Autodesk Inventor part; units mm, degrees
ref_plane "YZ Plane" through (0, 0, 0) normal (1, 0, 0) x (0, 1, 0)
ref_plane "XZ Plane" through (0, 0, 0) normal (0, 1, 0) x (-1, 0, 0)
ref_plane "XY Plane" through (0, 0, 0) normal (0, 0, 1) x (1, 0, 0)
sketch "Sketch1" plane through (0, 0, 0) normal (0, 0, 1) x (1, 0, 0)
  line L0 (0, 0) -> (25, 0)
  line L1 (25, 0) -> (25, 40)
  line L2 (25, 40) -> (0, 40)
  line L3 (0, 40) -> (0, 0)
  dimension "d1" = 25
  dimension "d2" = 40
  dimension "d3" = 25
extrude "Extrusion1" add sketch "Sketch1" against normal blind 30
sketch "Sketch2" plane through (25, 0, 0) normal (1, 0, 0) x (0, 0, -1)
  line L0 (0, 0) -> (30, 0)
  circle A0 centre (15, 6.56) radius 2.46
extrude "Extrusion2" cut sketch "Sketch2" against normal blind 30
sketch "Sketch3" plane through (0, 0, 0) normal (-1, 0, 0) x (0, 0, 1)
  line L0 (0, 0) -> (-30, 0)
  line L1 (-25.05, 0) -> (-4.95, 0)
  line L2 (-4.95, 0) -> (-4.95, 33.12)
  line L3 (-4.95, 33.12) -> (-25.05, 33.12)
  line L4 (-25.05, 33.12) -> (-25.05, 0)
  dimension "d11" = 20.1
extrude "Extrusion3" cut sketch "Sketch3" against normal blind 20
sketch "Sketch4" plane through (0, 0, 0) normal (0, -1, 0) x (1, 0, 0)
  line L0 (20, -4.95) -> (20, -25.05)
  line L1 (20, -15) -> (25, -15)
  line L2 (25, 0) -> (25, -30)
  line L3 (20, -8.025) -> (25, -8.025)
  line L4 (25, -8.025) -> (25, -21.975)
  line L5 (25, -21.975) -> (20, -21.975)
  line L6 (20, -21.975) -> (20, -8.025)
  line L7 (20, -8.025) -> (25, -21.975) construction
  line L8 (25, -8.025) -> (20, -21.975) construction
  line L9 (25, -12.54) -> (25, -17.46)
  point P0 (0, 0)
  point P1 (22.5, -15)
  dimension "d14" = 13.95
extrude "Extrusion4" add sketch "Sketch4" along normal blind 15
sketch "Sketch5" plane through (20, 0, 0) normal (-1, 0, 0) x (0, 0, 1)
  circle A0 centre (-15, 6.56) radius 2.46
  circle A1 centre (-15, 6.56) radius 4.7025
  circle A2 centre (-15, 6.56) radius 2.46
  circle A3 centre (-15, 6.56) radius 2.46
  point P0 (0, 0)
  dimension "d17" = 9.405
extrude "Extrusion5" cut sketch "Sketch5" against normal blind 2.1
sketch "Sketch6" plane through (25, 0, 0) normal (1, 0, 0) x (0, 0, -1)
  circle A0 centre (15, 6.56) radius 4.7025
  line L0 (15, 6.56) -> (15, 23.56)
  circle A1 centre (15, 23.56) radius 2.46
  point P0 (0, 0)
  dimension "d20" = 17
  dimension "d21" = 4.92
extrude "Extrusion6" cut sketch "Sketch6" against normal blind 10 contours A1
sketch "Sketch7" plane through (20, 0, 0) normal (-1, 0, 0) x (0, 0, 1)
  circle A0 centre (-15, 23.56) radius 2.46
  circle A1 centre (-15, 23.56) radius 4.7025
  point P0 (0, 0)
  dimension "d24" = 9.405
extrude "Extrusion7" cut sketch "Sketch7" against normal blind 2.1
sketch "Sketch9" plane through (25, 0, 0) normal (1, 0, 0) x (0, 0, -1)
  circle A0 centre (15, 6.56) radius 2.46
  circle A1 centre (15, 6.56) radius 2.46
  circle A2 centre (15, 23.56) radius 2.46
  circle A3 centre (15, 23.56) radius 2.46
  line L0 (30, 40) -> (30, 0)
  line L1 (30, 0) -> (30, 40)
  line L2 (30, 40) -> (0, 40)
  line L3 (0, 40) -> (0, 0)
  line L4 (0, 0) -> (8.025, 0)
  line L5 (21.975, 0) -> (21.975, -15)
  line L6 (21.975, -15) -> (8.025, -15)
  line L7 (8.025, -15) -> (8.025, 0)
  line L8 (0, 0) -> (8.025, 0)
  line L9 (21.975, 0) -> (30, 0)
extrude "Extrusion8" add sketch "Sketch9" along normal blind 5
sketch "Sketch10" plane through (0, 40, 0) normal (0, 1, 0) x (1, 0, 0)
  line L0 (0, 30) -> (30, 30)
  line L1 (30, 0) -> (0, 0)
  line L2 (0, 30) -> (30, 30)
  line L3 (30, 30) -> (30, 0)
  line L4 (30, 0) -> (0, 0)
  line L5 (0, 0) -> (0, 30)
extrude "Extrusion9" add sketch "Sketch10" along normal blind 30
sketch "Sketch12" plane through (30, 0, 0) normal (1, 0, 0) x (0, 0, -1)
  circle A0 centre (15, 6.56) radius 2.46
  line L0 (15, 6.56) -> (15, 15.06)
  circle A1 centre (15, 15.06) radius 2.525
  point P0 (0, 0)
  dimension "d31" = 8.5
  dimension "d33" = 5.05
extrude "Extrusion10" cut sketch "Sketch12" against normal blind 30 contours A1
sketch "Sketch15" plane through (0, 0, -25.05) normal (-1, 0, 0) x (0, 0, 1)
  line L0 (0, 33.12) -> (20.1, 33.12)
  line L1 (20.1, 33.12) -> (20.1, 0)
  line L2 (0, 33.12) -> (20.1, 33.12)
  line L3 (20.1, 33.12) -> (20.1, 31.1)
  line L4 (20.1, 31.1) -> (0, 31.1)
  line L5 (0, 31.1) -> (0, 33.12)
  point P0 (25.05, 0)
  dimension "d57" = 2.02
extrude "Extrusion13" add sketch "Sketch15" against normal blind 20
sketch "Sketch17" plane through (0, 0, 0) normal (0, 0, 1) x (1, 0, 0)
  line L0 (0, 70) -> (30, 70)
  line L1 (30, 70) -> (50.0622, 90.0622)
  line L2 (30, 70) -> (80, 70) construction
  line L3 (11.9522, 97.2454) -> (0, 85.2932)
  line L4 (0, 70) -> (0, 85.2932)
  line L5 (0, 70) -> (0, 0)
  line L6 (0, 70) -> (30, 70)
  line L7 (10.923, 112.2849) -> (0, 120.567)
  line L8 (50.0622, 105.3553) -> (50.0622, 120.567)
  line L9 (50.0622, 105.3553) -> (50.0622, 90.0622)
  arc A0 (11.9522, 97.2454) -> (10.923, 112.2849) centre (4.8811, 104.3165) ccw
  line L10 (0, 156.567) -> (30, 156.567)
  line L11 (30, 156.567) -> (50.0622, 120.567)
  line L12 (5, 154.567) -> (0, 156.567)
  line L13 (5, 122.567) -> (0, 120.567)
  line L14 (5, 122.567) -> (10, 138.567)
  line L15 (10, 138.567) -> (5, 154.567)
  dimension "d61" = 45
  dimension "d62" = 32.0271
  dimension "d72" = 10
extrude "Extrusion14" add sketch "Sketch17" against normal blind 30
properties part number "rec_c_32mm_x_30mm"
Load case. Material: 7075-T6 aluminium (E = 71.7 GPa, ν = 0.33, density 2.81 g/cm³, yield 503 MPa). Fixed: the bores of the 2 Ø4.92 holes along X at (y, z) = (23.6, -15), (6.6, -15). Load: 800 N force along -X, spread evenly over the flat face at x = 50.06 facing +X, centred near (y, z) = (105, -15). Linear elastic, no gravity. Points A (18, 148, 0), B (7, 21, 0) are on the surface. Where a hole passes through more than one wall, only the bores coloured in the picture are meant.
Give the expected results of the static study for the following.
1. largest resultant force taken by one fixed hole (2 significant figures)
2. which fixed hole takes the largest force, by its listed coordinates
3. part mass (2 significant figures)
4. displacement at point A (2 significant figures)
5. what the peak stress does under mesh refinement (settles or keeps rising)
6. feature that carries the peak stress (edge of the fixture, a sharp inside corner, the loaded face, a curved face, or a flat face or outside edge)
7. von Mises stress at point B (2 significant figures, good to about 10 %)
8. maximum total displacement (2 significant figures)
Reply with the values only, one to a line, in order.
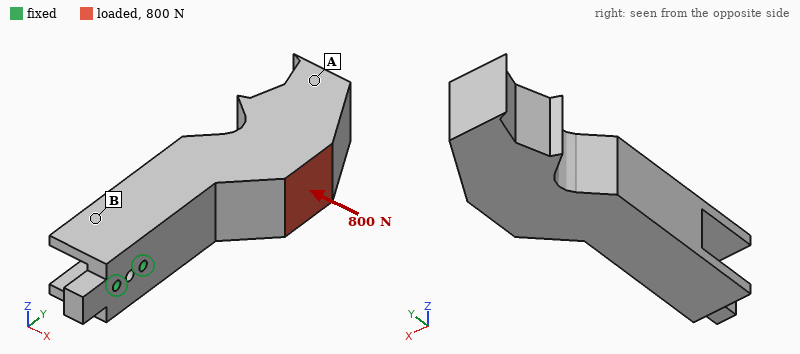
3.4 kN
(23.6, -15)
420 g
0.22 mm
keeps rising
edge of the fixture
17 MPa
0.24 mm
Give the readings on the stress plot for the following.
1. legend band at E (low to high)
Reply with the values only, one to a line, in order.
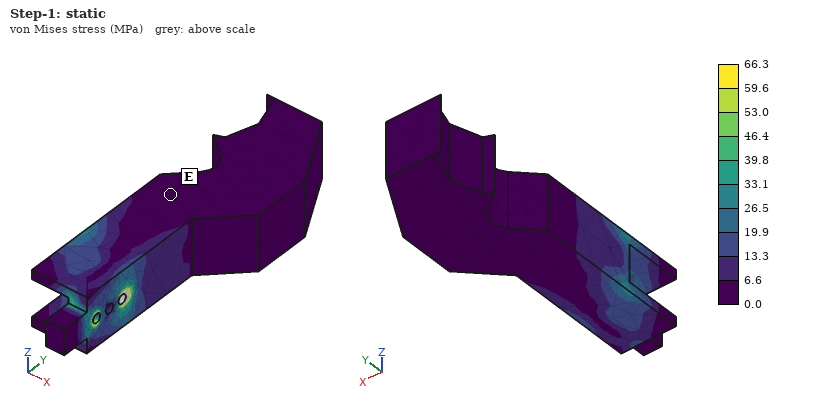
0.0 to 6.6 MPa
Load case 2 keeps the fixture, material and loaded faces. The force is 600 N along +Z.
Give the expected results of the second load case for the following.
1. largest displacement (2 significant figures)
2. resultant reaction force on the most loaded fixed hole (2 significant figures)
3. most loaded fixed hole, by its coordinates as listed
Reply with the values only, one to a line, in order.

0.16 mm
2.7 kN
(23.6, -15)
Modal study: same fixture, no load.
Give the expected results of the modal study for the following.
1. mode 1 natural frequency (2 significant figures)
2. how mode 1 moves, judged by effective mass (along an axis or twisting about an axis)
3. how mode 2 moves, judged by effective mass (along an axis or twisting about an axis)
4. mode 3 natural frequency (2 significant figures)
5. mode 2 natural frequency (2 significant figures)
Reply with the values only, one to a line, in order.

630 Hz
along X
along Z
2300 Hz
730 Hz
